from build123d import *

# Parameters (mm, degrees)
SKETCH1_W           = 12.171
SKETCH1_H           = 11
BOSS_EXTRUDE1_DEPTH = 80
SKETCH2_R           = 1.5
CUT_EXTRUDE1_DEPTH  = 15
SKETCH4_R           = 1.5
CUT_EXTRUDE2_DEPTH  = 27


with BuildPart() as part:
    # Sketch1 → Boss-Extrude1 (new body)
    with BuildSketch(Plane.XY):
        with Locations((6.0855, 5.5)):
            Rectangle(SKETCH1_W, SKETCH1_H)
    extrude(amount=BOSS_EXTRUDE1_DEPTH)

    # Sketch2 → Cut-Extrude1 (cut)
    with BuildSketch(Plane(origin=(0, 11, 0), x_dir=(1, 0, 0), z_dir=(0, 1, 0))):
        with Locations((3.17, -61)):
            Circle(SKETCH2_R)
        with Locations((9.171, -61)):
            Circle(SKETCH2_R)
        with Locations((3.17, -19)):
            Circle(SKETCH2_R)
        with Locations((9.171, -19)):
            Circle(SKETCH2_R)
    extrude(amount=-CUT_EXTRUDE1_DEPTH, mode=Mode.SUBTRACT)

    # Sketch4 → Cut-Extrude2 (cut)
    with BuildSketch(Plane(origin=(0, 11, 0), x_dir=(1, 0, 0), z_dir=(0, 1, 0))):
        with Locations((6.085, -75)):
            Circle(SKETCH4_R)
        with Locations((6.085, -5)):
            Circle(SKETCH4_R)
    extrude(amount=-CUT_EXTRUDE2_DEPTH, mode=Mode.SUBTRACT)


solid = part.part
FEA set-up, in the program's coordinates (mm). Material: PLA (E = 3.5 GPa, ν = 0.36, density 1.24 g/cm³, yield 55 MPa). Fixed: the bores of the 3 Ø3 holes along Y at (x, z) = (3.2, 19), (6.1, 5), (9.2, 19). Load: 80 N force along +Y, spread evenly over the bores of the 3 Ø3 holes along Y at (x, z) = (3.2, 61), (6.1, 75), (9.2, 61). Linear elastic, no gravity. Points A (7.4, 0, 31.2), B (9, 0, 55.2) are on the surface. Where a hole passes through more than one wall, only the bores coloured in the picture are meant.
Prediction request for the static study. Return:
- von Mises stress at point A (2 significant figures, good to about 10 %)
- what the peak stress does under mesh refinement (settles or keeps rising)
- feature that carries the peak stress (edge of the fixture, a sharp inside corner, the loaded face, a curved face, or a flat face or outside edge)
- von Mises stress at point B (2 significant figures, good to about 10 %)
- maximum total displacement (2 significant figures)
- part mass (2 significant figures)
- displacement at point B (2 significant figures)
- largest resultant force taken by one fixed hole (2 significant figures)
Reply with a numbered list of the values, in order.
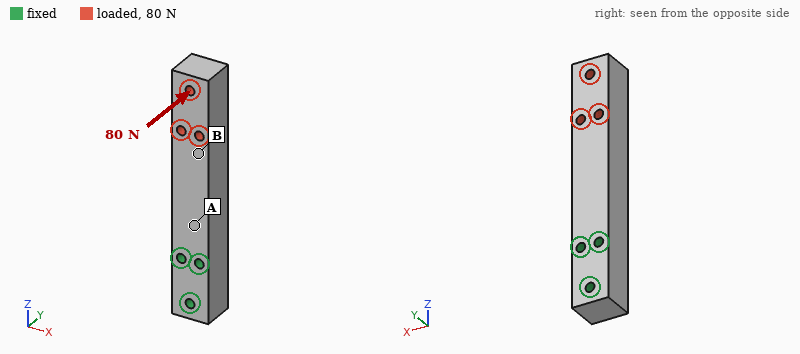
1. 11 MPa
2. keeps rising
3. edge of the fixture
4. 3.3 MPa
5. 0.84 mm
6. 13 g
7. 0.39 mm
8. 45 N
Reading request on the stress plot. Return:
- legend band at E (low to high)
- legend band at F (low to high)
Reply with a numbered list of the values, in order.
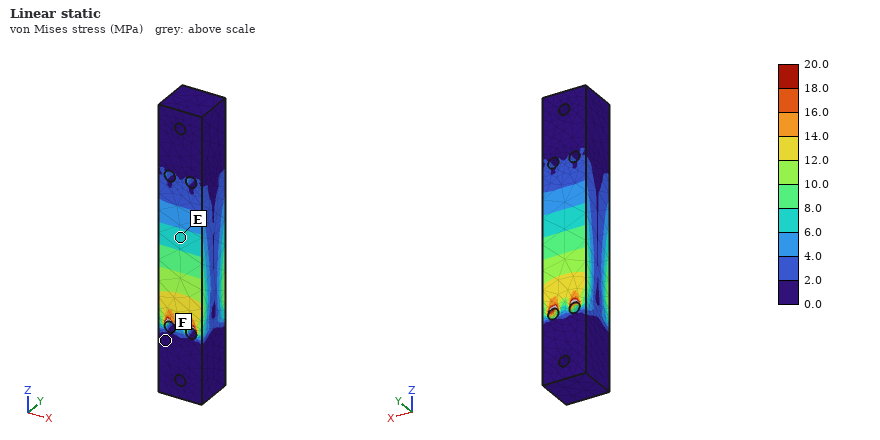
1. 6.0 to 8.0 MPa
2. 0.0 to 2.0 MPa
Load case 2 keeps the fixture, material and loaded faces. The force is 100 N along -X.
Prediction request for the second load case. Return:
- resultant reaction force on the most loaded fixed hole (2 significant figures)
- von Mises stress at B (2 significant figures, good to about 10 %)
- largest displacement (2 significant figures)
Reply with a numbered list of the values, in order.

1. 570 N
2. 2.5 MPa
3. 0.89 mm
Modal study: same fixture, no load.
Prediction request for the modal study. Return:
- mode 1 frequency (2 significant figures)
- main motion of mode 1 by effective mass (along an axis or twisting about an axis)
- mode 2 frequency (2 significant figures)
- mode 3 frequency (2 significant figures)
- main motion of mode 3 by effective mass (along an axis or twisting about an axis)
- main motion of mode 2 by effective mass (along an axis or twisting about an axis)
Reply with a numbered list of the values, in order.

1. 830 Hz
2. along Y
3. 890 Hz
4. 3900 Hz
5. twisting about Z
6. along X
